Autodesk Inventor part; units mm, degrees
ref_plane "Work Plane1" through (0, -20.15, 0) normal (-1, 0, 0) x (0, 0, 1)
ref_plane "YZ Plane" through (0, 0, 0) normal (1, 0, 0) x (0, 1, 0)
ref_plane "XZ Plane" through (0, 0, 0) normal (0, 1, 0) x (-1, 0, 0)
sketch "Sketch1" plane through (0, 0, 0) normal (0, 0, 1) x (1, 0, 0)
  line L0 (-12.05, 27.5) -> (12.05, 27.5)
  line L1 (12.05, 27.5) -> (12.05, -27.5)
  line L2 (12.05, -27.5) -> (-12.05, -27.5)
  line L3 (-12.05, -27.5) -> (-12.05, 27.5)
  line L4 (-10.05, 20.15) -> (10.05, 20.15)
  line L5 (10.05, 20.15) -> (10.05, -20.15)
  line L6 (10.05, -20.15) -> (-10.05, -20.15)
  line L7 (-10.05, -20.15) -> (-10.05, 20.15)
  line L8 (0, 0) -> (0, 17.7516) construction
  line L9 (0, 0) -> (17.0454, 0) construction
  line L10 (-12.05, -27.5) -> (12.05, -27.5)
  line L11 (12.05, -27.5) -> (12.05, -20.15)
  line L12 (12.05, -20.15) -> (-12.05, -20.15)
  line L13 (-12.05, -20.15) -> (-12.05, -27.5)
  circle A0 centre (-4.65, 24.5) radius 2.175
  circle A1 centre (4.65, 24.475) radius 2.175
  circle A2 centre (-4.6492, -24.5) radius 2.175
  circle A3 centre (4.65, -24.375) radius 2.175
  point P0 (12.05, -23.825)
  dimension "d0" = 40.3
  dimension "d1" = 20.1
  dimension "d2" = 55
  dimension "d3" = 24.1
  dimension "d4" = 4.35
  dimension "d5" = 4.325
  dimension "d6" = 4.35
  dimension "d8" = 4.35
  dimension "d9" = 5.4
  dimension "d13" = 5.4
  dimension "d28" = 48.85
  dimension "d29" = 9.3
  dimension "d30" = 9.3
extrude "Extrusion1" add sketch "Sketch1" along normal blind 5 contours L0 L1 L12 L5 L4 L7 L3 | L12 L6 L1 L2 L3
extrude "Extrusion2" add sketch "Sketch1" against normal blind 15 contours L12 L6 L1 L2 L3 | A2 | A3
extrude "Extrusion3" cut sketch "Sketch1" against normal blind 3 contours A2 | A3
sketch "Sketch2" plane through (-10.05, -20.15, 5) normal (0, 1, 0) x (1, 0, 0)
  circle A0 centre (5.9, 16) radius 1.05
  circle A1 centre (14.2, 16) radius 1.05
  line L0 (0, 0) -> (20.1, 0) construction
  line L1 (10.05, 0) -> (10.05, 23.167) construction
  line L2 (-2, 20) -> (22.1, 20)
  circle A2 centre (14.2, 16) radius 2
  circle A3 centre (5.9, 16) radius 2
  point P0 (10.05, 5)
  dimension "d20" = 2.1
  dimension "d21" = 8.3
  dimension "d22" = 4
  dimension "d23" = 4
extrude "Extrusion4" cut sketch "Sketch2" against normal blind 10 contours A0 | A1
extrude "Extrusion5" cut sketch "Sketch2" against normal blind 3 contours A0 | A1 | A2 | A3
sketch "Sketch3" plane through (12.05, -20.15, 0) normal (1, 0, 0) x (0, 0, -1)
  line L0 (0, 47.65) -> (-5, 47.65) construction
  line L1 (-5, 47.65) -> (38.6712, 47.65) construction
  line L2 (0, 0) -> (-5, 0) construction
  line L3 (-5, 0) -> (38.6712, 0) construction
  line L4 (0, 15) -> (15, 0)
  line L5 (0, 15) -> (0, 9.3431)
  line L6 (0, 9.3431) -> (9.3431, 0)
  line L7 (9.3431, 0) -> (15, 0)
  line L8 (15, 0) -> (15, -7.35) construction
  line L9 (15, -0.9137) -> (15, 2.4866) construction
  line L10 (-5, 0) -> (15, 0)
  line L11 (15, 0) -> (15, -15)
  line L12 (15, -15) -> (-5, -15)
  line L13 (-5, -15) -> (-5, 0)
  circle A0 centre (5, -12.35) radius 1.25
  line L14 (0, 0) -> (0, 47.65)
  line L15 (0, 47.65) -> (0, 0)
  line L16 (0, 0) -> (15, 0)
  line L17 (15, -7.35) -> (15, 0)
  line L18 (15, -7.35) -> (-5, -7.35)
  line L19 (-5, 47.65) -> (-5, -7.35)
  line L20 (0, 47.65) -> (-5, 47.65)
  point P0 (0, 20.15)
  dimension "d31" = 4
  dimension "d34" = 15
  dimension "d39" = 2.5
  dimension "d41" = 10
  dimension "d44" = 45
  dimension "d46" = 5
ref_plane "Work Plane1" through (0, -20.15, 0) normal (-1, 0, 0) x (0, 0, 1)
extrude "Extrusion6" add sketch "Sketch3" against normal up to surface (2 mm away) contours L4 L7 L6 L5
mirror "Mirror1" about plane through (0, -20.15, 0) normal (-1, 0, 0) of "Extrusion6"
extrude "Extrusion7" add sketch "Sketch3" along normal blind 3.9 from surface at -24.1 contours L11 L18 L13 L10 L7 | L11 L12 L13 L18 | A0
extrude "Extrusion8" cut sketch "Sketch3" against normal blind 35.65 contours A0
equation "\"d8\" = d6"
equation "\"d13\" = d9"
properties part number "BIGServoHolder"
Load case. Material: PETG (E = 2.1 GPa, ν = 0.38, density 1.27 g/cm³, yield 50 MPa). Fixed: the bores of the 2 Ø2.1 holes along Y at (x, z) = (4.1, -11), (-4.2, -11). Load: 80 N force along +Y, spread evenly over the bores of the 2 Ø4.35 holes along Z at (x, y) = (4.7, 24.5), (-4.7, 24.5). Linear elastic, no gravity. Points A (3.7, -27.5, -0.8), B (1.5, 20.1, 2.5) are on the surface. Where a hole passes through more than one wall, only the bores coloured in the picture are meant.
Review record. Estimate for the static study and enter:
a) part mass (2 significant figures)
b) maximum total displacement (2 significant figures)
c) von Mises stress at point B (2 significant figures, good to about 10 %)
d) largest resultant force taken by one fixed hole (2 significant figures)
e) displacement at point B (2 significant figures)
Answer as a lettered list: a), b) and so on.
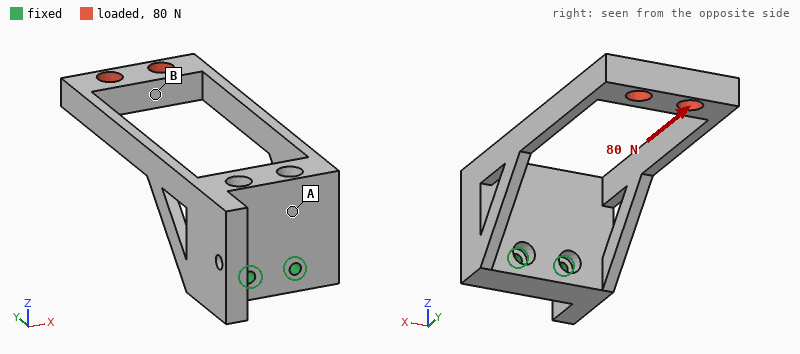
a) 7.1 g
b) 0.74 mm
c) 7.8 MPa
d) 40 N
e) 0.63 mm
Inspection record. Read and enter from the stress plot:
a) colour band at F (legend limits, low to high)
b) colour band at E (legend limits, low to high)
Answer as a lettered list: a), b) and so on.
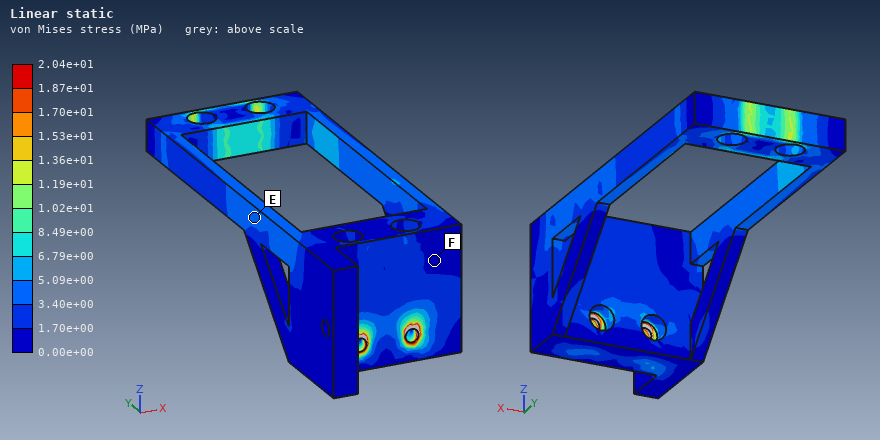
a) 0.00e+00 to 1.70e+00 MPa
b) 3.40e+00 to 5.09e+00 MPa
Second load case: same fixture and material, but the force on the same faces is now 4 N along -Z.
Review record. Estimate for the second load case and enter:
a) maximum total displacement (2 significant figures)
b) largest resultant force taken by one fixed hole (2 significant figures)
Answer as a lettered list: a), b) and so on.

a) 0.81 mm
b) 3.5 N
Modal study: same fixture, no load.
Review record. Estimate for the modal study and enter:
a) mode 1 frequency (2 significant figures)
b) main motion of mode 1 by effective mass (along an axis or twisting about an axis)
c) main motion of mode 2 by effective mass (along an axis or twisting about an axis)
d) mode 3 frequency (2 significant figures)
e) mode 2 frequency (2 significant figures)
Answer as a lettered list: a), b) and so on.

a) 230 Hz
b) along X
c) along Z
d) 920 Hz
e) 370 Hz
